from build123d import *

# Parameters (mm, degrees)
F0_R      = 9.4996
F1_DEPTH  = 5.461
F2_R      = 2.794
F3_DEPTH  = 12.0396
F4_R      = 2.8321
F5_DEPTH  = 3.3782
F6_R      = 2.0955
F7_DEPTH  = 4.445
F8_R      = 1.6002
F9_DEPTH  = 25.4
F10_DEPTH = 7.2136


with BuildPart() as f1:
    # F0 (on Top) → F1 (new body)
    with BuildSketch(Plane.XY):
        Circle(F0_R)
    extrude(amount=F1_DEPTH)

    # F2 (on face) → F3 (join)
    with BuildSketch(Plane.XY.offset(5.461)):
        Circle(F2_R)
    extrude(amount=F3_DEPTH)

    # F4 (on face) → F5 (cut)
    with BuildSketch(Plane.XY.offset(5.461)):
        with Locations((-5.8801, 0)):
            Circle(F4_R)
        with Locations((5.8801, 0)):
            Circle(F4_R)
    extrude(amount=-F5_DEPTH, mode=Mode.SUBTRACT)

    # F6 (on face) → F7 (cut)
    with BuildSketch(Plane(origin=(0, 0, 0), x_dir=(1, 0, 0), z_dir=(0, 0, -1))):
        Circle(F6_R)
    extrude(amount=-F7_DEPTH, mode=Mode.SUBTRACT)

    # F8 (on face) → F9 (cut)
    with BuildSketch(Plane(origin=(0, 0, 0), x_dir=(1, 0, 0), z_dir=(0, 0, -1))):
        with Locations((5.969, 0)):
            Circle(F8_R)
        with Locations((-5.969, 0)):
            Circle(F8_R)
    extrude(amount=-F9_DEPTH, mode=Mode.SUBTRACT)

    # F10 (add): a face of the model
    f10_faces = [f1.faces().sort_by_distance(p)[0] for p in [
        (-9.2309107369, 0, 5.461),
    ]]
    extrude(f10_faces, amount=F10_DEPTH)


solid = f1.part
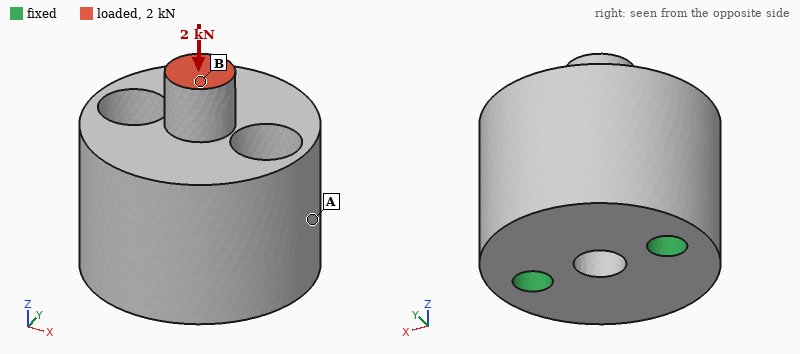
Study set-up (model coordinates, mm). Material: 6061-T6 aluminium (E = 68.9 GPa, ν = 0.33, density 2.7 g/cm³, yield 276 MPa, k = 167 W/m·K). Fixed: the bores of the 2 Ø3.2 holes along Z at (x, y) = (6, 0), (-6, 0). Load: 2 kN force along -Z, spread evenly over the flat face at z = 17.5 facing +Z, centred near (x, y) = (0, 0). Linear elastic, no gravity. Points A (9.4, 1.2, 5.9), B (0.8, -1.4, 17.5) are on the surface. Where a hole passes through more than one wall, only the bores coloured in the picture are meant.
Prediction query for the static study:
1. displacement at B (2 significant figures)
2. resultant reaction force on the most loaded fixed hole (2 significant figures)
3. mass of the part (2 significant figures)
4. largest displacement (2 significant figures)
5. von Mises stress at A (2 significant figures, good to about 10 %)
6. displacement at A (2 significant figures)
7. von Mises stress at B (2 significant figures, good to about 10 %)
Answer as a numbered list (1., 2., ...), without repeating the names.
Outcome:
1. 15 µm
2. 1.0 kN
3. 8.3 g
4. 15 µm
5. 23 MPa
6. 3.7 µm
7. 82 MPa
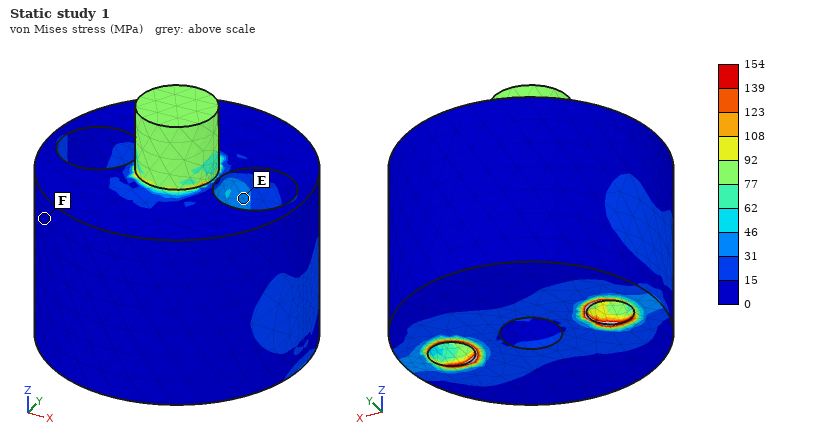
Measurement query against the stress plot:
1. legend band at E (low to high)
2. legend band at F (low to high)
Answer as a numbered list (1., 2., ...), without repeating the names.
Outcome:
1. 31 to 46 MPa
2. 0 to 15 MPa
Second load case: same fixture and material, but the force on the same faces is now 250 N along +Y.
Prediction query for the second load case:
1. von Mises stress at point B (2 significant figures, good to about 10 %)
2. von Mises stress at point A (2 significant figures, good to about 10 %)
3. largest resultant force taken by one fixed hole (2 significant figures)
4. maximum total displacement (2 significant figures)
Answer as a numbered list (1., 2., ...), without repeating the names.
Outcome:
1. 23 MPa
2. 18 MPa
3. 130 N
4. 44 µm
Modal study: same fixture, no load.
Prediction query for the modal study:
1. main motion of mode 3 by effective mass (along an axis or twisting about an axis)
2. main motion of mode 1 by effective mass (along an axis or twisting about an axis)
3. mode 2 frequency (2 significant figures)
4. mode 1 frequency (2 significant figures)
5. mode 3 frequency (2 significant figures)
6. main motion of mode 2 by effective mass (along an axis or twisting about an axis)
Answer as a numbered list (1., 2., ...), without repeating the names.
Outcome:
1. along Z
2. along Y
3. 23 kHz
4. 8900 Hz
5. 34 kHz
6. along X
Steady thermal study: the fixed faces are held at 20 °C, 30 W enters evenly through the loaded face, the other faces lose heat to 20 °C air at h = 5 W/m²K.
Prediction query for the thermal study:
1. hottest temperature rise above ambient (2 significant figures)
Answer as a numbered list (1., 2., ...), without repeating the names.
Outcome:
1. 63 K
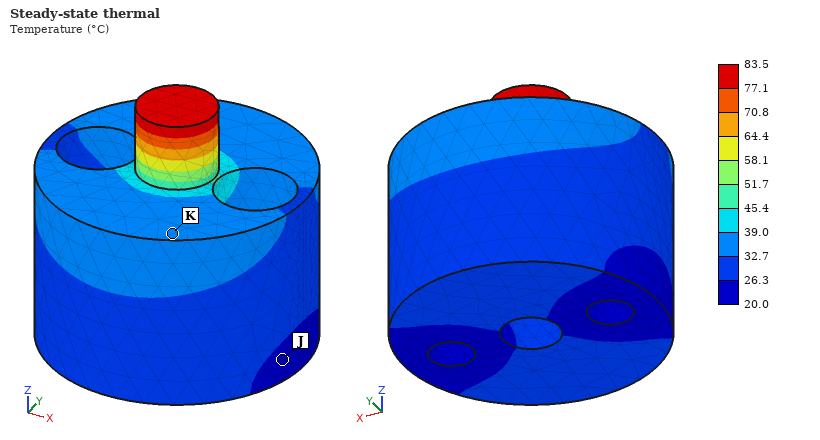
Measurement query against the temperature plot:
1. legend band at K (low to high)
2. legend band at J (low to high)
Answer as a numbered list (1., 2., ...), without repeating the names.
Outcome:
1. 32.7 to 39.0 °C
2. 20.0 to 26.3 °C
